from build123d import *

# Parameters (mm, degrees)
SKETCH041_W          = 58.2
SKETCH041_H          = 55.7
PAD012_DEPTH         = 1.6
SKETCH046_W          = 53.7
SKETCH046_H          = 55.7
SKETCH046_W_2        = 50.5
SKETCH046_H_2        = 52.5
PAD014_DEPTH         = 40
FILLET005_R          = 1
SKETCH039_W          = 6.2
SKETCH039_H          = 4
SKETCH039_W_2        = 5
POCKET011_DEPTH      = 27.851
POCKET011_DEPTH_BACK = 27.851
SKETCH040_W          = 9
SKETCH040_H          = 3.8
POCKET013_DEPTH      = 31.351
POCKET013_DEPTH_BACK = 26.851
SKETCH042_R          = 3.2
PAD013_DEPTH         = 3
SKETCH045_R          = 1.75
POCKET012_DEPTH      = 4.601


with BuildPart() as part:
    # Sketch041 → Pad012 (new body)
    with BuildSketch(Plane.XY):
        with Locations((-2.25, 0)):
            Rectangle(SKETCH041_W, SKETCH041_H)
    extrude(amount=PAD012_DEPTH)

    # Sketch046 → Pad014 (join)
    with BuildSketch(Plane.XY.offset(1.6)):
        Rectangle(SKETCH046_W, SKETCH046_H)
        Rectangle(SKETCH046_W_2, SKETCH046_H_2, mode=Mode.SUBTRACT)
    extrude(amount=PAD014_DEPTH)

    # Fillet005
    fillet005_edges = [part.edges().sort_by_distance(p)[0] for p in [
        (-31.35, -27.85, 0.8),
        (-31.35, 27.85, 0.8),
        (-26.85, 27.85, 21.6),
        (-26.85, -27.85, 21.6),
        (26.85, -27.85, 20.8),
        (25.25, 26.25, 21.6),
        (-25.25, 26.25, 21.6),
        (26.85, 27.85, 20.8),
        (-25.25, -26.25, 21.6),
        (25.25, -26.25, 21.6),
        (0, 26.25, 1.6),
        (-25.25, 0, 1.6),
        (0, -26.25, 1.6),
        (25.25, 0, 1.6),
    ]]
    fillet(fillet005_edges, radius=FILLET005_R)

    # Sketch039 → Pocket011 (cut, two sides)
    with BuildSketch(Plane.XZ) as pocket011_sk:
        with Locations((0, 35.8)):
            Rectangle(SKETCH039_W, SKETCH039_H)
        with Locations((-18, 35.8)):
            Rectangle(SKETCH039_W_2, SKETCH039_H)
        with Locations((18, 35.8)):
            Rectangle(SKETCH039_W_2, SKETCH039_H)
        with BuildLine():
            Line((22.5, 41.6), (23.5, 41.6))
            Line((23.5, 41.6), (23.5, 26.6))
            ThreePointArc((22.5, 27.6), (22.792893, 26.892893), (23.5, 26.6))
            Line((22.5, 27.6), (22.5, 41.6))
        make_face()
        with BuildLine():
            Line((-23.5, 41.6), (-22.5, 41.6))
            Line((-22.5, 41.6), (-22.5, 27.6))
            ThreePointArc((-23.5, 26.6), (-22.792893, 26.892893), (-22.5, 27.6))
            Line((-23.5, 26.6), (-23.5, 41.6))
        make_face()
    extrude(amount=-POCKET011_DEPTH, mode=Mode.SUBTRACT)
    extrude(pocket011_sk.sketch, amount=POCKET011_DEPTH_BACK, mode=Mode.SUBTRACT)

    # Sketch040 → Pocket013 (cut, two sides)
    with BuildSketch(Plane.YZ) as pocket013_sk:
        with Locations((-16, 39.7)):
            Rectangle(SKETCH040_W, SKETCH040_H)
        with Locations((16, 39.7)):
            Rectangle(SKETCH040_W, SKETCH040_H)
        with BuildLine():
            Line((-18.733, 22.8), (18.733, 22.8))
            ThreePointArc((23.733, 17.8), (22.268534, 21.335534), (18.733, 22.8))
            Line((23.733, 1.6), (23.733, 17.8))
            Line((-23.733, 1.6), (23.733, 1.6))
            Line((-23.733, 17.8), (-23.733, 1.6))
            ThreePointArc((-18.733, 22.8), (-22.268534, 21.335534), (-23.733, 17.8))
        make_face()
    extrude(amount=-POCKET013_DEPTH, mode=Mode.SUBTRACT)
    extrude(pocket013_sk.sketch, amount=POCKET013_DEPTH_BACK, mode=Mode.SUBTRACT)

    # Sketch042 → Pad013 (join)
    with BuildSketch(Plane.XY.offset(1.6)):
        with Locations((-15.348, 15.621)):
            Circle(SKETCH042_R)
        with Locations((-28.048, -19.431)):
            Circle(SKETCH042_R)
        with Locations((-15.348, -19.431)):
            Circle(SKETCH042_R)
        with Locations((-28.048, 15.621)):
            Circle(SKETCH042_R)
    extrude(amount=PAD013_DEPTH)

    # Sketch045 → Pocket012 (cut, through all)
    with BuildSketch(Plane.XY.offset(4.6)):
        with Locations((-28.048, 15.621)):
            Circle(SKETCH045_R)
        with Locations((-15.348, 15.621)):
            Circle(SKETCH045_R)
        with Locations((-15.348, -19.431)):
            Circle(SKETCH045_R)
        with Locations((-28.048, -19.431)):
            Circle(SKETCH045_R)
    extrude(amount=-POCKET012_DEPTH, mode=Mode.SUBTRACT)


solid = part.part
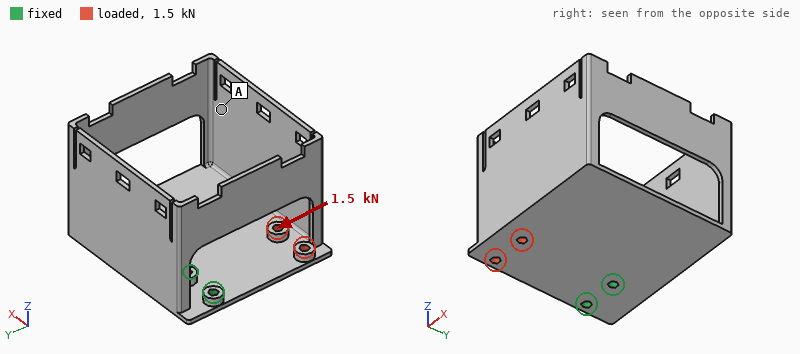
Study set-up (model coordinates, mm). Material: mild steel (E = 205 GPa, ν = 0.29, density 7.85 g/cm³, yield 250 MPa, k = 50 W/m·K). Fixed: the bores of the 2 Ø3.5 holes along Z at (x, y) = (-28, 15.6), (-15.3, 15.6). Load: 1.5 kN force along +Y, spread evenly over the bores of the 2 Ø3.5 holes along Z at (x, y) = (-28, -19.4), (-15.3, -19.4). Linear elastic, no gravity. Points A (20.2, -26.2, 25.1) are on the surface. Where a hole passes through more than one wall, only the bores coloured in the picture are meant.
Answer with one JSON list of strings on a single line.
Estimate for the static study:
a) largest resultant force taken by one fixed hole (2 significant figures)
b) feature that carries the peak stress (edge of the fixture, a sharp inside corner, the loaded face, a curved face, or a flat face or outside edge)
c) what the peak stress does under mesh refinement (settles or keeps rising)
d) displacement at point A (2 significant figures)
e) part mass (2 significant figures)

["760 N", "a sharp inside corner", "keeps rising", "0.29 mm", "120 g"]
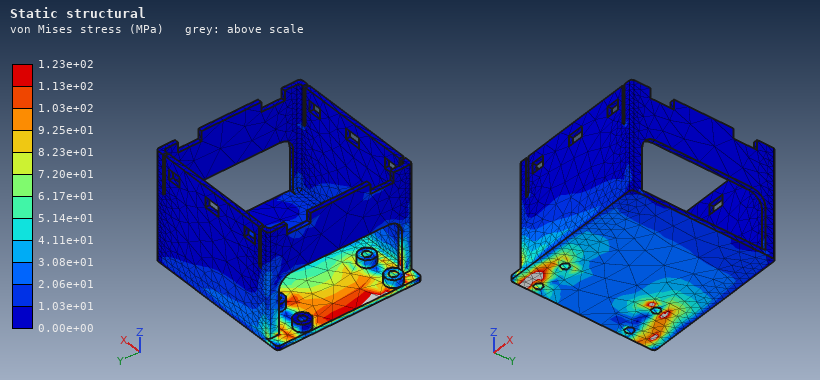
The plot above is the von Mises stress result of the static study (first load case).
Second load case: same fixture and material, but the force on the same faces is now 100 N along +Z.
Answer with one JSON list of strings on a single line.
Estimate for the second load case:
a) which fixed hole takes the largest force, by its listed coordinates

["(-28, 15.6)"]
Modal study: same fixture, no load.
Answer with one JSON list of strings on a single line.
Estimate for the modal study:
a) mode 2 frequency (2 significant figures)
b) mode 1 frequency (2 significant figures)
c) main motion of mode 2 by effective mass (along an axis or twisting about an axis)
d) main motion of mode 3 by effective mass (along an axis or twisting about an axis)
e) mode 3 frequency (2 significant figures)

["480 Hz", "280 Hz", "along X", "along Z", "820 Hz"]
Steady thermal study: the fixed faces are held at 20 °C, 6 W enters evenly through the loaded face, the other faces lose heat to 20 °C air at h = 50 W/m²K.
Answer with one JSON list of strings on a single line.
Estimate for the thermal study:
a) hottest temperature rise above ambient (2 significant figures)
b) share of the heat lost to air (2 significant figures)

["37 K", "79 %"]
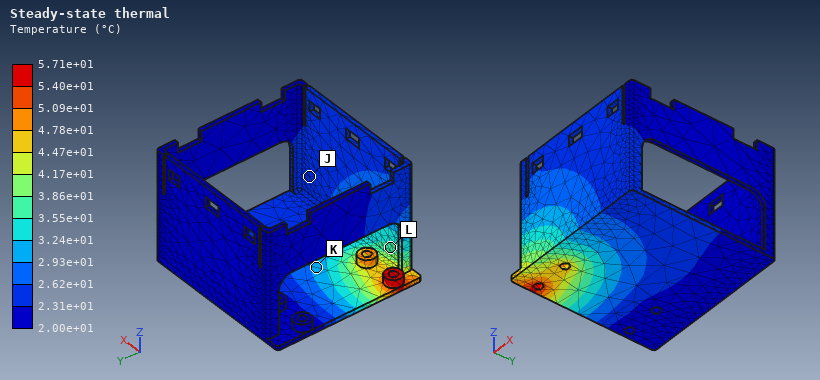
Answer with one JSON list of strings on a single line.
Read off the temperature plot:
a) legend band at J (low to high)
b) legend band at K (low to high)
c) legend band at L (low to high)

["2.31e+01 to 2.62e+01 °C", "2.93e+01 to 3.24e+01 °C", "3.55e+01 to 3.86e+01 °C"]
